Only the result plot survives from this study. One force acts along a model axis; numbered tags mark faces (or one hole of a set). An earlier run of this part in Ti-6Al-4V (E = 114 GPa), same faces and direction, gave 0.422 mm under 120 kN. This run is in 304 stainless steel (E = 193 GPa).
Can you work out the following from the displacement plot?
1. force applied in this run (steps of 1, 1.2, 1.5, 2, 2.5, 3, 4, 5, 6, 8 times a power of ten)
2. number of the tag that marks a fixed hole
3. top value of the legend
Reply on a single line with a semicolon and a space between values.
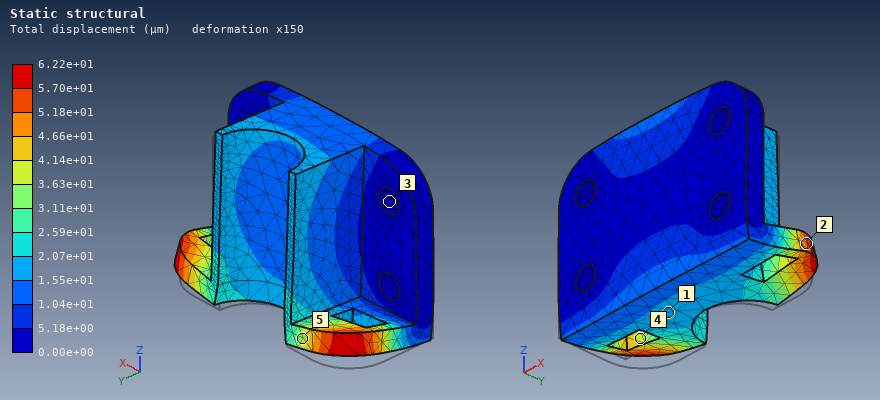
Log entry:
30 kN; 3; 6.22e+01 µm
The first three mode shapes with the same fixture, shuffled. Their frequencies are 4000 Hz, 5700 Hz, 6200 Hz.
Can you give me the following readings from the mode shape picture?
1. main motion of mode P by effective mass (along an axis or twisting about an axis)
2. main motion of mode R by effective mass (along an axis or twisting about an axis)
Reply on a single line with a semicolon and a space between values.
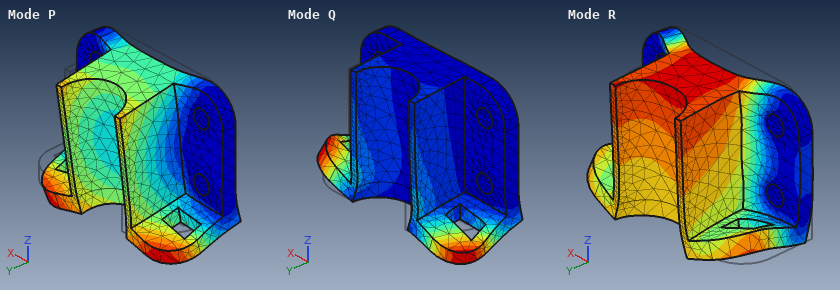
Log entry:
along Z; along Y
